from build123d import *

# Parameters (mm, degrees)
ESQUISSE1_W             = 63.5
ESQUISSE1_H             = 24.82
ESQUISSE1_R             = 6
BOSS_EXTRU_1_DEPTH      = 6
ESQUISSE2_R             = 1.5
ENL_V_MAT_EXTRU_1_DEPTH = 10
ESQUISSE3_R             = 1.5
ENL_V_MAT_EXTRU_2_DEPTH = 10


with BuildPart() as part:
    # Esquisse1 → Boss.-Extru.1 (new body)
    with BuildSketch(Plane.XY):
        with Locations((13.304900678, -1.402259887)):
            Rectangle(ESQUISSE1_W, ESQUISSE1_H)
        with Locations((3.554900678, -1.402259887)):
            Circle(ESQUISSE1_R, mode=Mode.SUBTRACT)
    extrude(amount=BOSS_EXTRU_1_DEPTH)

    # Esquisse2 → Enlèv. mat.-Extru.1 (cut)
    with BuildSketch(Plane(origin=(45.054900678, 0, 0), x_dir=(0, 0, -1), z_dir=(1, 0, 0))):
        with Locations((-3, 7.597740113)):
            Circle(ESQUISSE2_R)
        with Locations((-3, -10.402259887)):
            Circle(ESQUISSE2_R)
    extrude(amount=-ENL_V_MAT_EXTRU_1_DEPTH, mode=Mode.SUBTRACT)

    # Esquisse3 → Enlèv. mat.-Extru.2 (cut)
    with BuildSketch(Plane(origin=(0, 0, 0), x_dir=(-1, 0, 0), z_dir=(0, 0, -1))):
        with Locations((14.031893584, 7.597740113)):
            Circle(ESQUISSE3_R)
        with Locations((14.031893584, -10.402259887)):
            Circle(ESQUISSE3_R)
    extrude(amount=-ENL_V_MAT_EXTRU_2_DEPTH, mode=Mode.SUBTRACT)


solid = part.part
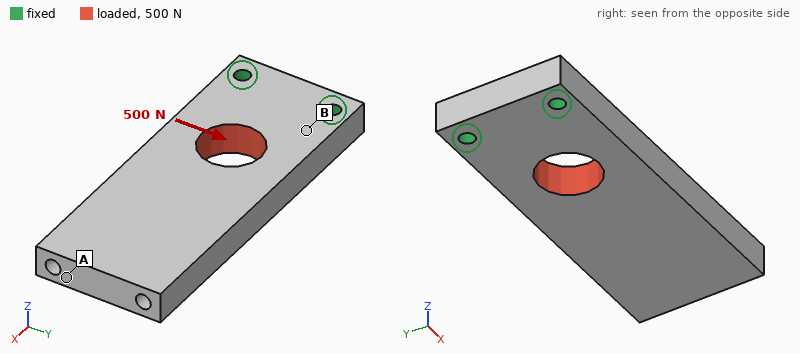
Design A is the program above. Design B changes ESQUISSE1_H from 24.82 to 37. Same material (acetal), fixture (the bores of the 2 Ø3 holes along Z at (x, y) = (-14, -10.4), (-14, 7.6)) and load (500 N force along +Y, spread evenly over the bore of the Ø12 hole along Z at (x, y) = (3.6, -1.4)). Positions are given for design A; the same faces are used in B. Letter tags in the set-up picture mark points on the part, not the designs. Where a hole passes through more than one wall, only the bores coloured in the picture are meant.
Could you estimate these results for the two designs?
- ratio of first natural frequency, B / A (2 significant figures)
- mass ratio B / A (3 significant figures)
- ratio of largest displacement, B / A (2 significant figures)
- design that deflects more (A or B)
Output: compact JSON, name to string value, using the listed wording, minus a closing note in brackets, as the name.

{"ratio of first natural frequency, B / A": "1.0", "mass ratio B / A": "1.54", "ratio of largest displacement, B / A": "0.72", "design that deflects more": "A"}
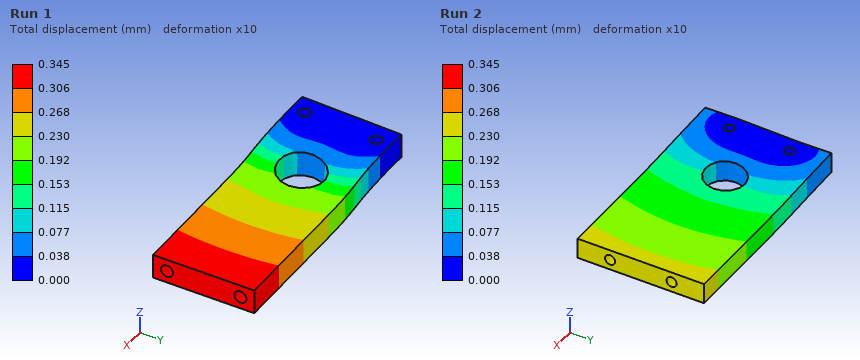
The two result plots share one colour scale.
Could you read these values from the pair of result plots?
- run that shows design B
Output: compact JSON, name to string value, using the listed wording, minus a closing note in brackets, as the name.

{"run that shows design B": "Run 2"}
